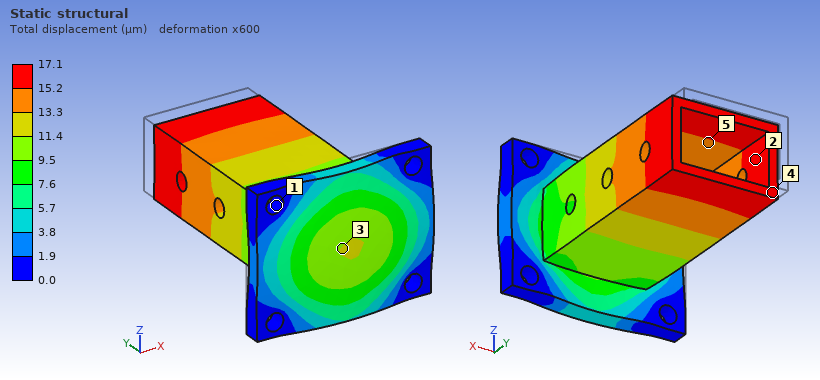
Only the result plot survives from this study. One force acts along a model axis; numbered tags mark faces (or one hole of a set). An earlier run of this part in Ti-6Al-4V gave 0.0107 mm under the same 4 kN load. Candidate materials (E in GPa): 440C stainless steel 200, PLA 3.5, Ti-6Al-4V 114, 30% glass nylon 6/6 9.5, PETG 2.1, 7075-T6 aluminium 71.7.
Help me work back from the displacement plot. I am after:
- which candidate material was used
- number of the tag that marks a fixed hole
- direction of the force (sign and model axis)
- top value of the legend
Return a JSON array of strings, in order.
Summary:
["7075-T6 aluminium", "1", "-Y", "17.1 µm"]
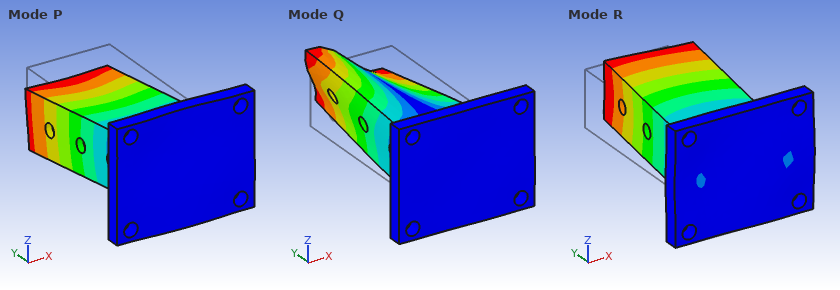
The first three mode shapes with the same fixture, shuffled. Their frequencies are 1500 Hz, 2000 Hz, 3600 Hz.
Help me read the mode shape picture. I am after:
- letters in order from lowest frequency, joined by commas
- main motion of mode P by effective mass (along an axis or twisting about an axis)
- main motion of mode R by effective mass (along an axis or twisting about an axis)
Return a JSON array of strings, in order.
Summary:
["P, R, Q", "along Z", "along X"]
